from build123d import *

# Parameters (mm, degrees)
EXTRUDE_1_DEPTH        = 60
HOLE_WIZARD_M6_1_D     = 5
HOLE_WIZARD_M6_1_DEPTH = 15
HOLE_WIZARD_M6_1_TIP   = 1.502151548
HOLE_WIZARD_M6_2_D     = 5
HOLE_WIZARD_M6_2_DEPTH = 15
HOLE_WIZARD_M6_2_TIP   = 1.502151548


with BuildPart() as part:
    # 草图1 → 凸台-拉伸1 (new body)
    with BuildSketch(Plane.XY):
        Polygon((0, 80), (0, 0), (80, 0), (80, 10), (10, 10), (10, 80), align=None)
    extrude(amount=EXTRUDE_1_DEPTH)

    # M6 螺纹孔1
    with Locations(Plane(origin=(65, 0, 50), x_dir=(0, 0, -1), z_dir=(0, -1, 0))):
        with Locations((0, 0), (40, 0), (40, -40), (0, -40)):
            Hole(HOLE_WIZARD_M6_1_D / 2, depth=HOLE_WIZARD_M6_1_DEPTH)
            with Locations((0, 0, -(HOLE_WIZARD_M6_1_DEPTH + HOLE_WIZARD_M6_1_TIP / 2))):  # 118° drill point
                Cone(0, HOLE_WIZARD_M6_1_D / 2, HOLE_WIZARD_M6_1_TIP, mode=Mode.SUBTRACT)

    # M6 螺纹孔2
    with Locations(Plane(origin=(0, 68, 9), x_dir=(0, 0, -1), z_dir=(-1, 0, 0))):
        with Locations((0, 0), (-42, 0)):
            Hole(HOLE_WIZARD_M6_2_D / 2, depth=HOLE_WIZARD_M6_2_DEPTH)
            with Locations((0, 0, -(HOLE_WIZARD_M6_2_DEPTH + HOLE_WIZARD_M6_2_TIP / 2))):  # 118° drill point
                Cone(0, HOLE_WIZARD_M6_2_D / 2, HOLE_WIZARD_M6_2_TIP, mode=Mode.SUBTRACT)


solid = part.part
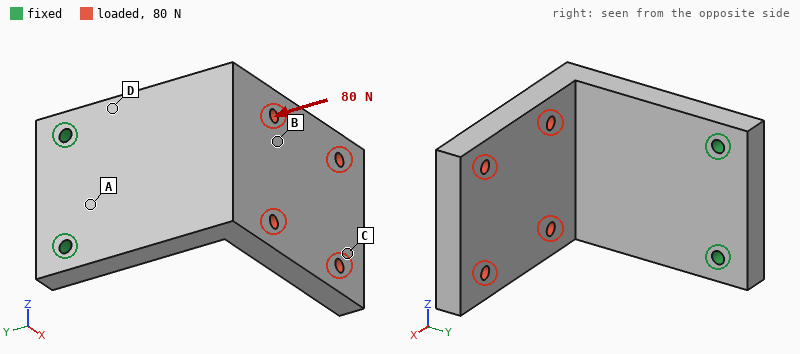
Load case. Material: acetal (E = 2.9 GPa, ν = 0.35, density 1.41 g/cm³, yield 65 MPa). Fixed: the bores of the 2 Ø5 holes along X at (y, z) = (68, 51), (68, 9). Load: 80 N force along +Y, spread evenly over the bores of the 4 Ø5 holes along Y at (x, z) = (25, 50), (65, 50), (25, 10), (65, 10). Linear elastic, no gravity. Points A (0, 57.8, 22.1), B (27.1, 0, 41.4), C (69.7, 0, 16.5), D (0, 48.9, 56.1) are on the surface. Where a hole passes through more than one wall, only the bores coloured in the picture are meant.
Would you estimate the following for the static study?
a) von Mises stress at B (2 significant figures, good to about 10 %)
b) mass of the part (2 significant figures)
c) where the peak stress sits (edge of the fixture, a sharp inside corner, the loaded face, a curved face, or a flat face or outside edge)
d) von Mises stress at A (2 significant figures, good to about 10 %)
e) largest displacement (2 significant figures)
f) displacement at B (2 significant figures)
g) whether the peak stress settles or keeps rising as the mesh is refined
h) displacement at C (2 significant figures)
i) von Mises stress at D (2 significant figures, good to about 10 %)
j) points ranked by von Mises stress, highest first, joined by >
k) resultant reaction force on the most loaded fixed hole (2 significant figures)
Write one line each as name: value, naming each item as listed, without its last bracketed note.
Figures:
von Mises stress at B: 1.5 MPa
mass of the part: 130 g
where the peak stress sits: edge of the fixture
von Mises stress at A: 2.4 MPa
largest displacement: 1.4 mm
displacement at B: 0.65 mm
whether the peak stress settles or keeps rising as the mesh is refined: keeps rising
displacement at C: 1.3 mm
von Mises stress at D: 3.2 MPa
points ranked by von Mises stress, highest first, joined by >: D > A > B > C
resultant reaction force on the most loaded fixed hole: 41 N
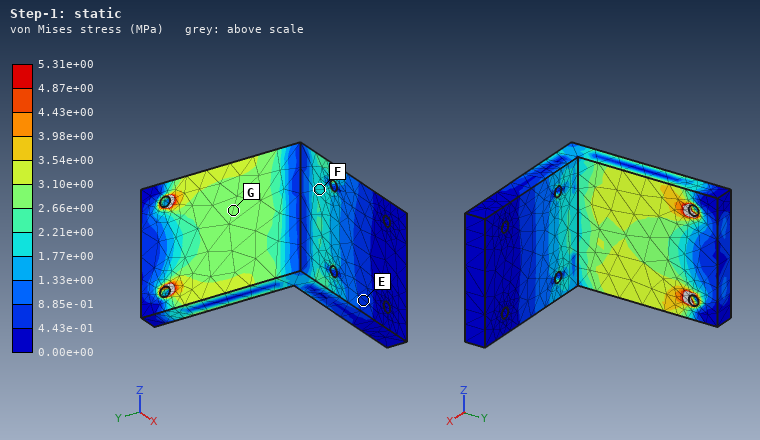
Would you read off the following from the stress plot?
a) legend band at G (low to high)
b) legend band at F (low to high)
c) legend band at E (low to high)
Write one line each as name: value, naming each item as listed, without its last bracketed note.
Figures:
legend band at G: 2.66e+00 to 3.10e+00 MPa
legend band at F: 1.77e+00 to 2.21e+00 MPa
legend band at E: 4.43e-01 to 8.85e-01 MPa
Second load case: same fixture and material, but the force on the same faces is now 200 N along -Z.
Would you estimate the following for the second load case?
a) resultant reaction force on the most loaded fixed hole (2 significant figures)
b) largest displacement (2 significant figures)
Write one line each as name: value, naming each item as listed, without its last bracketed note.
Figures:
resultant reaction force on the most loaded fixed hole: 350 N
largest displacement: 1.5 mm
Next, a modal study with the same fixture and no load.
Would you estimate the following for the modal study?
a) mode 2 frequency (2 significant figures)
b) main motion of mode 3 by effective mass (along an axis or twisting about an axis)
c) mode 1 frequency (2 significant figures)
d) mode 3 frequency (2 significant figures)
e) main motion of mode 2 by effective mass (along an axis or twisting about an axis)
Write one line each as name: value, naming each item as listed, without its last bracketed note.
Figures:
mode 2 frequency: 280 Hz
main motion of mode 3 by effective mass: along X
mode 1 frequency: 160 Hz
mode 3 frequency: 440 Hz
main motion of mode 2 by effective mass: along Z
